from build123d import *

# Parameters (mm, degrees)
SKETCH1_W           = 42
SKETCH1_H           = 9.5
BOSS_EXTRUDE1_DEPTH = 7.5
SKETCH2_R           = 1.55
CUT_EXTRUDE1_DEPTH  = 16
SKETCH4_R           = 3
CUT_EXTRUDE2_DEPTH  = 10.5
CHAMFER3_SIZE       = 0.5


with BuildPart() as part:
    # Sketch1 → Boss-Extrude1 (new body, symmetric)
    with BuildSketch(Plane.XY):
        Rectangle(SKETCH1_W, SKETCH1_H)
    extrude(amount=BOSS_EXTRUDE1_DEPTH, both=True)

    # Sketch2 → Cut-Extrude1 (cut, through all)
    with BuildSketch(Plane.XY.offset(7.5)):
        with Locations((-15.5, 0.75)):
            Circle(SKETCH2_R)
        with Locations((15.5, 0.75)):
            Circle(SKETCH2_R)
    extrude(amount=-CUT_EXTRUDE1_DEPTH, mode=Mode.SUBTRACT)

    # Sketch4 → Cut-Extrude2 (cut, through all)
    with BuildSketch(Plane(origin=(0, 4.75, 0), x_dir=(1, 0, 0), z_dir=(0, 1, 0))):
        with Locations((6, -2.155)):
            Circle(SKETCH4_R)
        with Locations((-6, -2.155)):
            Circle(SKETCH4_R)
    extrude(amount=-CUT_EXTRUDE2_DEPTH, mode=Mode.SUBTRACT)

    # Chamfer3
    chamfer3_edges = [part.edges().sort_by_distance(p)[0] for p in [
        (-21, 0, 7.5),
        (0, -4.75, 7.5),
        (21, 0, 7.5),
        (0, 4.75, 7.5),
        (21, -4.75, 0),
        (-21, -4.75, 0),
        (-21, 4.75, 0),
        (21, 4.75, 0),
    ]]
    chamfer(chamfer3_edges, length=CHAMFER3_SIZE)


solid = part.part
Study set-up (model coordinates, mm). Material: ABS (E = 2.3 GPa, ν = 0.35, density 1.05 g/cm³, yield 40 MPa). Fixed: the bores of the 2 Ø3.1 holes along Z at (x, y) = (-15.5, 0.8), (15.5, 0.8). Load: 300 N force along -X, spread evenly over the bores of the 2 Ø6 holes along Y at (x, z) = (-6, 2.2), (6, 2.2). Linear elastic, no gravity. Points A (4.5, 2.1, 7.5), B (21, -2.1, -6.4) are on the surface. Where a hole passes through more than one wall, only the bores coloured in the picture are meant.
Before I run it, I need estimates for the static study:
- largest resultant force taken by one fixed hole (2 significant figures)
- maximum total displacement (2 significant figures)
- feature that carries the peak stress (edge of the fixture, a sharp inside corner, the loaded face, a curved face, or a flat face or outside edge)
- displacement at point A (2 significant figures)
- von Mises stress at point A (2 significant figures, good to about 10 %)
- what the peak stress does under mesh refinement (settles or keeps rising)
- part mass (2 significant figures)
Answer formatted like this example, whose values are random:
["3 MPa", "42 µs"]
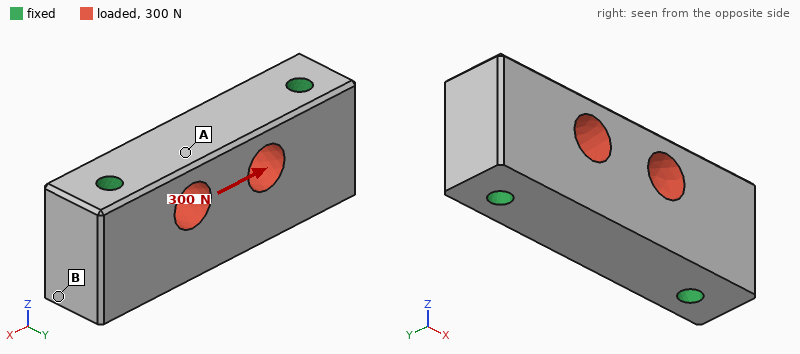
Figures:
["150 N", "11 µm", "edge of the fixture", "6.9 µm", "0.89 MPa", "keeps rising", "5.5 g"]
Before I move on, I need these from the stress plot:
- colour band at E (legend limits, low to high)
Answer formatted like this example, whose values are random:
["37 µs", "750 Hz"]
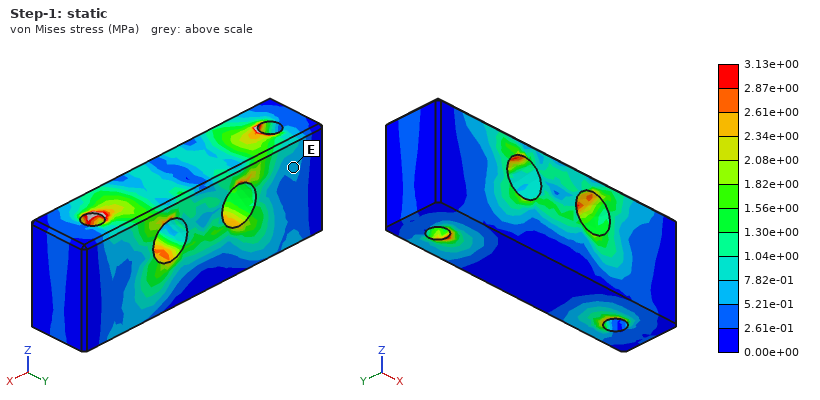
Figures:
["5.21e-01 to 7.82e-01 MPa"]
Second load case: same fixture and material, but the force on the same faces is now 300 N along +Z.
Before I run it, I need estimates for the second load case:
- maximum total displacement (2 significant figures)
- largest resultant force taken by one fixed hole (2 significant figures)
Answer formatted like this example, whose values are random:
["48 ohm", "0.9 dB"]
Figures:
["28 µm", "150 N"]
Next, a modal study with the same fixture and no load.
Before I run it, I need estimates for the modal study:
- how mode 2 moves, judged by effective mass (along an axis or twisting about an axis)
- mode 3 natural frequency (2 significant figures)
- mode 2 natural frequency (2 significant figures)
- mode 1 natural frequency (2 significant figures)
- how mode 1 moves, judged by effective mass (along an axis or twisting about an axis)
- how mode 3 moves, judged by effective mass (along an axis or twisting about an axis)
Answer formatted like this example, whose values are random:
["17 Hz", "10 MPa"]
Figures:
["along Z", "12 kHz", "11 kHz", "8600 Hz", "along Y", "twisting about X"]
